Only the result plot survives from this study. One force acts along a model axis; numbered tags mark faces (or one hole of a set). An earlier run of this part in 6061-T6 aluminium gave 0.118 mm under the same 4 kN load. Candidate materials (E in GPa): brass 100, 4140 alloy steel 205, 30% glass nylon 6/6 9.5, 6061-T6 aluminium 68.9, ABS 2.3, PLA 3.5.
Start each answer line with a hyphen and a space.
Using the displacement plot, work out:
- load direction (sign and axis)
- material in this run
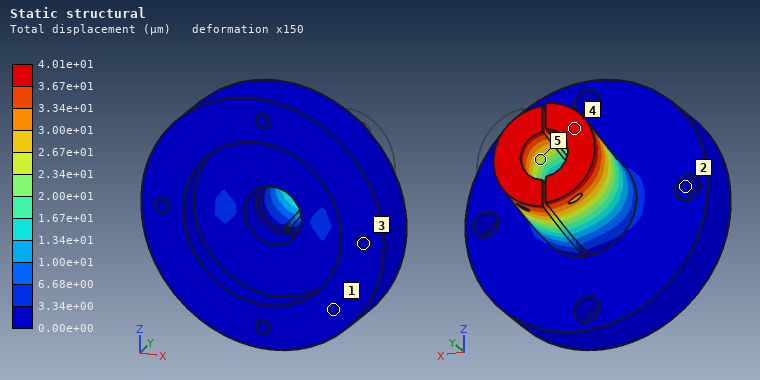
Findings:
- -X
- 4140 alloy steel
